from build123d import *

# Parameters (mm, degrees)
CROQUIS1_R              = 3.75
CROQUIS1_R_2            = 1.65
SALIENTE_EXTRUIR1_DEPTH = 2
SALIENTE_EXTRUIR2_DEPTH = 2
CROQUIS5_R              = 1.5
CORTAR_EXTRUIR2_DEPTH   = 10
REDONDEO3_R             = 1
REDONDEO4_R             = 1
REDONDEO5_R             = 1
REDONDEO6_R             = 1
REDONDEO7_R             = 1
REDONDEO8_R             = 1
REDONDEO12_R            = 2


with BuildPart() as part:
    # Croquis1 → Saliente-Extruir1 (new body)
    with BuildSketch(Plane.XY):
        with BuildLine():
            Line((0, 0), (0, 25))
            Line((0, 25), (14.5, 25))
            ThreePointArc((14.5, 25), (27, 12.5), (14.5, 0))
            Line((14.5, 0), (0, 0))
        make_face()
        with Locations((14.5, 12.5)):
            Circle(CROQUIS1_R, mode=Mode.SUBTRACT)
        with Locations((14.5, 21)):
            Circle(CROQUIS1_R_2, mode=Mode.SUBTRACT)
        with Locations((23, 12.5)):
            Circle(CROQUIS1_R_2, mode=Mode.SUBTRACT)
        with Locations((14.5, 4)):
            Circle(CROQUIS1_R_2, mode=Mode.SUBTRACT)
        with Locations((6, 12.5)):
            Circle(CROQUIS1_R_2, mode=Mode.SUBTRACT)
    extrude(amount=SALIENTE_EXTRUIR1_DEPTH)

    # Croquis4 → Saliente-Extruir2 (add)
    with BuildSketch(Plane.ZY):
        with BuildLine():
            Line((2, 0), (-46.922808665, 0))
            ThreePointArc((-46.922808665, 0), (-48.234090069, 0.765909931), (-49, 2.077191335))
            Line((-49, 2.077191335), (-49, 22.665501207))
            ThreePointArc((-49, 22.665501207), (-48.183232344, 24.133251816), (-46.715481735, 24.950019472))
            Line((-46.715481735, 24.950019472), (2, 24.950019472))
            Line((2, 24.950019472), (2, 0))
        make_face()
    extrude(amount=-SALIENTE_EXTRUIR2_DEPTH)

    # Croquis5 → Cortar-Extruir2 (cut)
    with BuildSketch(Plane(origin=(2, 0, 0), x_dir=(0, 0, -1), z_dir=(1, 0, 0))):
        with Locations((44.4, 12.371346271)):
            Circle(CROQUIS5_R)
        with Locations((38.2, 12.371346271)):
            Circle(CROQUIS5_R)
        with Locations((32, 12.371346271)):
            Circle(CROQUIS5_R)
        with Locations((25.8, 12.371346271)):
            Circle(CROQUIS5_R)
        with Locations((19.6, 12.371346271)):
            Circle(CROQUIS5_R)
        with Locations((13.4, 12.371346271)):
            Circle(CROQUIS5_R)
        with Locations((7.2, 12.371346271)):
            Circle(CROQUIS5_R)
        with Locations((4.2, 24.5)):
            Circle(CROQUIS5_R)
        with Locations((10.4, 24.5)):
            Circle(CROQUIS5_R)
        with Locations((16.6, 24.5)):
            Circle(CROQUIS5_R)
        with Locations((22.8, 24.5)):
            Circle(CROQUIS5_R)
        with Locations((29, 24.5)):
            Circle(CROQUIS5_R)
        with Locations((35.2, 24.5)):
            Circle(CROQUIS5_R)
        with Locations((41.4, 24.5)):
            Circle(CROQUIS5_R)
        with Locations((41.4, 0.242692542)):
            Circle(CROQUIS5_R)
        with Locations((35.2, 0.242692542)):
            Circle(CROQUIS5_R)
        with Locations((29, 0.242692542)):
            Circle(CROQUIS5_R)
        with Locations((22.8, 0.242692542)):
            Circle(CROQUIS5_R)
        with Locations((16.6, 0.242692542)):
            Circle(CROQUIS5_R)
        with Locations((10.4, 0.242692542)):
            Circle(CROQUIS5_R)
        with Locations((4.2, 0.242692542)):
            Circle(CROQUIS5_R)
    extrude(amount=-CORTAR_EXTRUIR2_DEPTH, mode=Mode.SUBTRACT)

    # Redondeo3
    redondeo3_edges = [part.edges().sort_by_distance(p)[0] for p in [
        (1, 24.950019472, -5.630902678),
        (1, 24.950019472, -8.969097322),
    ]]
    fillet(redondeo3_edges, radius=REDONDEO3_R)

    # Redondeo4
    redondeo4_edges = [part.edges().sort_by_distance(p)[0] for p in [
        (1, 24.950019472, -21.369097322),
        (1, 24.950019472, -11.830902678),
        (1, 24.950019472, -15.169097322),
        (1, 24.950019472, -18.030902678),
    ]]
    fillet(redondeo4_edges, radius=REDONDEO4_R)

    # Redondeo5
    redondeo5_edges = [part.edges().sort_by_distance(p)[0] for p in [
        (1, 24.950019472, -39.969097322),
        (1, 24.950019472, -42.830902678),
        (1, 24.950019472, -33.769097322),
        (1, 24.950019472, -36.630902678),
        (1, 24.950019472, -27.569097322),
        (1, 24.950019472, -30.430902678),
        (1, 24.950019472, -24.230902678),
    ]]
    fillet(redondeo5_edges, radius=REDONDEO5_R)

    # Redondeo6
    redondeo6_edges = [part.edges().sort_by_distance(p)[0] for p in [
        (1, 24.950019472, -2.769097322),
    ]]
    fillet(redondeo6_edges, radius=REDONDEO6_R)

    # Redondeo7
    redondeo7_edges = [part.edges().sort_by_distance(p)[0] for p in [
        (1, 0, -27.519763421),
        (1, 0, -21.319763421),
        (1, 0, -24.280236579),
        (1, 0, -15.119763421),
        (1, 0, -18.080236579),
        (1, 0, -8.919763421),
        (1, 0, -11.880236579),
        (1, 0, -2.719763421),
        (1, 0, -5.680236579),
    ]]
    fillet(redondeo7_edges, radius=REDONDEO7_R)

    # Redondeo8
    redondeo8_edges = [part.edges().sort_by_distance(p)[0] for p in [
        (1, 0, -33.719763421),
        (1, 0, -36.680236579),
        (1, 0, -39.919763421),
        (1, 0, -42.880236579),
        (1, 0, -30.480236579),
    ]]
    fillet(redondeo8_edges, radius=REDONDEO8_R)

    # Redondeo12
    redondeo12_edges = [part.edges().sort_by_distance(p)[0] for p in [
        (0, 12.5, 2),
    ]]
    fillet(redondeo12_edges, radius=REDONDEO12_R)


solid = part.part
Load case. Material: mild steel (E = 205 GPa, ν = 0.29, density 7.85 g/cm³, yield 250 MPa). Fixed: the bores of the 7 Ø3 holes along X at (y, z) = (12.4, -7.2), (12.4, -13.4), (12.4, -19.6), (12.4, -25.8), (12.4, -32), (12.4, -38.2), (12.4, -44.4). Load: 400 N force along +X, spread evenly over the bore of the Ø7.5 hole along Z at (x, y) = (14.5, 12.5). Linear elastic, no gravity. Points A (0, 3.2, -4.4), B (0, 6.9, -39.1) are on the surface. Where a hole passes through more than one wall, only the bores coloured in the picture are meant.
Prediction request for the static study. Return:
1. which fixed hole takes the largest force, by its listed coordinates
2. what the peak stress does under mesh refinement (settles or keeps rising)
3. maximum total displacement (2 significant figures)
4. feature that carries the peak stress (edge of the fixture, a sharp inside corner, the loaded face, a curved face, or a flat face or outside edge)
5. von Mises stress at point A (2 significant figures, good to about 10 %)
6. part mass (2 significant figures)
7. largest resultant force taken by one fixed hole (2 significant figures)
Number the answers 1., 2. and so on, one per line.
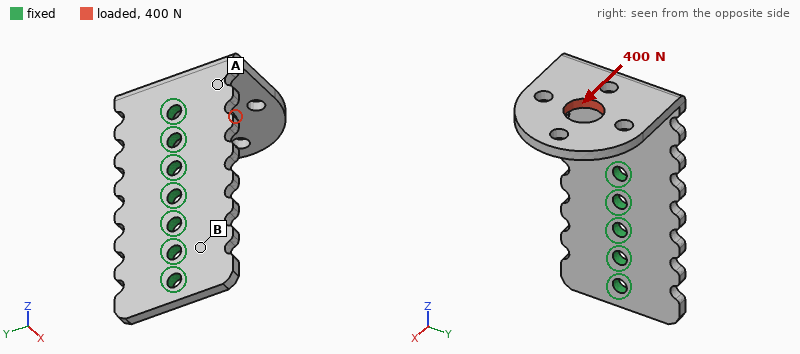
1. (12.4, -7.2)
2. keeps rising
3. 0.12 mm
4. edge of the fixture
5. 86 MPa
6. 25 g
7. 550 N
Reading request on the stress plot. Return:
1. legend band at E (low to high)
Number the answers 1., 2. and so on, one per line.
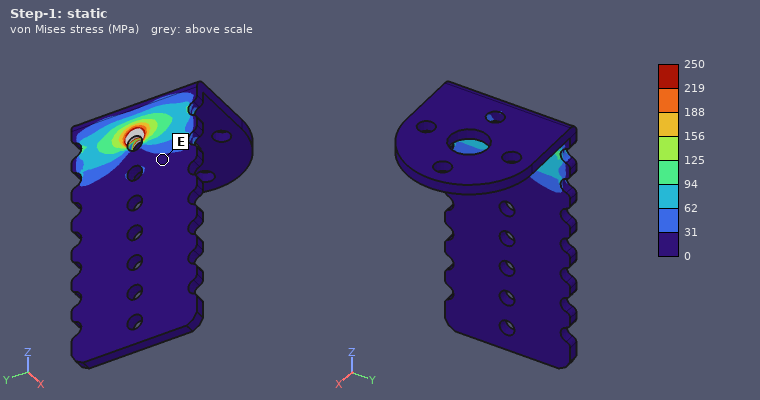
1. 0 to 31 MPa
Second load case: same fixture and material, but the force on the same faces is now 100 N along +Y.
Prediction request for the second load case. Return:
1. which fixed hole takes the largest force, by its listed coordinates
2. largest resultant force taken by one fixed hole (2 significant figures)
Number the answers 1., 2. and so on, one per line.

1. (12.4, -7.2)
2. 130 N
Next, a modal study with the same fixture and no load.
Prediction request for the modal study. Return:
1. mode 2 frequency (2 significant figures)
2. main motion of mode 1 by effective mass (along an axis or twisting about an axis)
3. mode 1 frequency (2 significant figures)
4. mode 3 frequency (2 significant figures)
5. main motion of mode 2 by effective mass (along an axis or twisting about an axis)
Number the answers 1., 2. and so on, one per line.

1. 2900 Hz
2. along Z
3. 1900 Hz
4. 6700 Hz
5. along Y
